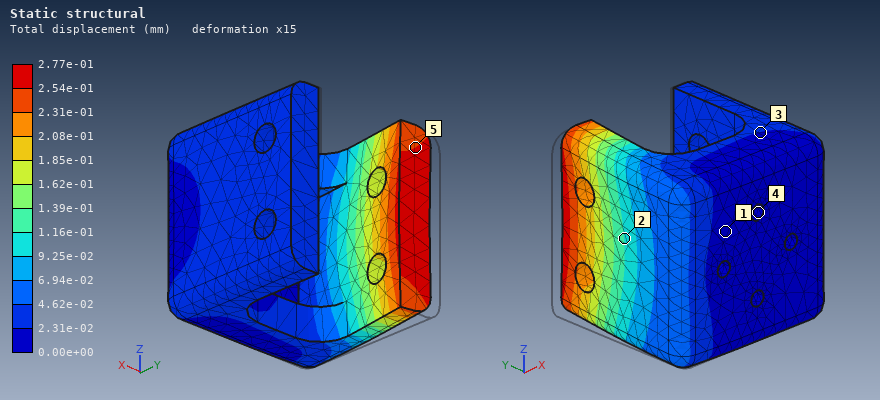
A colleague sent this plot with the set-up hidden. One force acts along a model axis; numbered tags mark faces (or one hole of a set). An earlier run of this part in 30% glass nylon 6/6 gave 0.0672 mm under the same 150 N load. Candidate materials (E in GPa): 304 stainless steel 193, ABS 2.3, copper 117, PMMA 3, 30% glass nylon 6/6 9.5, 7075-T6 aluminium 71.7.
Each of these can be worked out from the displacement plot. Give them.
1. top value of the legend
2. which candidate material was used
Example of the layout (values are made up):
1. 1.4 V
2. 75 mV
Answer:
1. 2.77e-01 mm
2. ABS
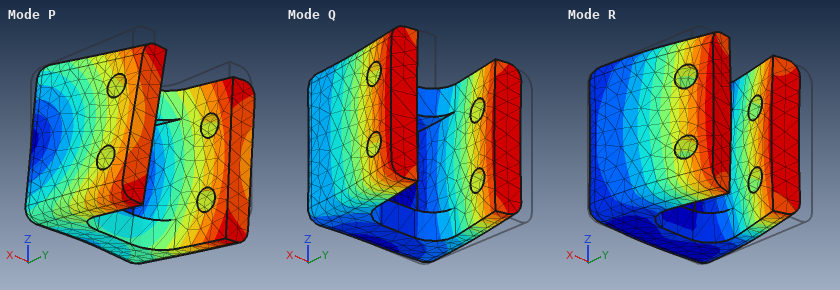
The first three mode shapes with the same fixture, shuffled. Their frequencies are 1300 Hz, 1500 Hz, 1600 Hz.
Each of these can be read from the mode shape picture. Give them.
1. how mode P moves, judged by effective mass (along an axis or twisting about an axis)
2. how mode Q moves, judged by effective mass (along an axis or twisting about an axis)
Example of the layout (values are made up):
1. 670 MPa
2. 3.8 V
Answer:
1. along Z
2. along X
